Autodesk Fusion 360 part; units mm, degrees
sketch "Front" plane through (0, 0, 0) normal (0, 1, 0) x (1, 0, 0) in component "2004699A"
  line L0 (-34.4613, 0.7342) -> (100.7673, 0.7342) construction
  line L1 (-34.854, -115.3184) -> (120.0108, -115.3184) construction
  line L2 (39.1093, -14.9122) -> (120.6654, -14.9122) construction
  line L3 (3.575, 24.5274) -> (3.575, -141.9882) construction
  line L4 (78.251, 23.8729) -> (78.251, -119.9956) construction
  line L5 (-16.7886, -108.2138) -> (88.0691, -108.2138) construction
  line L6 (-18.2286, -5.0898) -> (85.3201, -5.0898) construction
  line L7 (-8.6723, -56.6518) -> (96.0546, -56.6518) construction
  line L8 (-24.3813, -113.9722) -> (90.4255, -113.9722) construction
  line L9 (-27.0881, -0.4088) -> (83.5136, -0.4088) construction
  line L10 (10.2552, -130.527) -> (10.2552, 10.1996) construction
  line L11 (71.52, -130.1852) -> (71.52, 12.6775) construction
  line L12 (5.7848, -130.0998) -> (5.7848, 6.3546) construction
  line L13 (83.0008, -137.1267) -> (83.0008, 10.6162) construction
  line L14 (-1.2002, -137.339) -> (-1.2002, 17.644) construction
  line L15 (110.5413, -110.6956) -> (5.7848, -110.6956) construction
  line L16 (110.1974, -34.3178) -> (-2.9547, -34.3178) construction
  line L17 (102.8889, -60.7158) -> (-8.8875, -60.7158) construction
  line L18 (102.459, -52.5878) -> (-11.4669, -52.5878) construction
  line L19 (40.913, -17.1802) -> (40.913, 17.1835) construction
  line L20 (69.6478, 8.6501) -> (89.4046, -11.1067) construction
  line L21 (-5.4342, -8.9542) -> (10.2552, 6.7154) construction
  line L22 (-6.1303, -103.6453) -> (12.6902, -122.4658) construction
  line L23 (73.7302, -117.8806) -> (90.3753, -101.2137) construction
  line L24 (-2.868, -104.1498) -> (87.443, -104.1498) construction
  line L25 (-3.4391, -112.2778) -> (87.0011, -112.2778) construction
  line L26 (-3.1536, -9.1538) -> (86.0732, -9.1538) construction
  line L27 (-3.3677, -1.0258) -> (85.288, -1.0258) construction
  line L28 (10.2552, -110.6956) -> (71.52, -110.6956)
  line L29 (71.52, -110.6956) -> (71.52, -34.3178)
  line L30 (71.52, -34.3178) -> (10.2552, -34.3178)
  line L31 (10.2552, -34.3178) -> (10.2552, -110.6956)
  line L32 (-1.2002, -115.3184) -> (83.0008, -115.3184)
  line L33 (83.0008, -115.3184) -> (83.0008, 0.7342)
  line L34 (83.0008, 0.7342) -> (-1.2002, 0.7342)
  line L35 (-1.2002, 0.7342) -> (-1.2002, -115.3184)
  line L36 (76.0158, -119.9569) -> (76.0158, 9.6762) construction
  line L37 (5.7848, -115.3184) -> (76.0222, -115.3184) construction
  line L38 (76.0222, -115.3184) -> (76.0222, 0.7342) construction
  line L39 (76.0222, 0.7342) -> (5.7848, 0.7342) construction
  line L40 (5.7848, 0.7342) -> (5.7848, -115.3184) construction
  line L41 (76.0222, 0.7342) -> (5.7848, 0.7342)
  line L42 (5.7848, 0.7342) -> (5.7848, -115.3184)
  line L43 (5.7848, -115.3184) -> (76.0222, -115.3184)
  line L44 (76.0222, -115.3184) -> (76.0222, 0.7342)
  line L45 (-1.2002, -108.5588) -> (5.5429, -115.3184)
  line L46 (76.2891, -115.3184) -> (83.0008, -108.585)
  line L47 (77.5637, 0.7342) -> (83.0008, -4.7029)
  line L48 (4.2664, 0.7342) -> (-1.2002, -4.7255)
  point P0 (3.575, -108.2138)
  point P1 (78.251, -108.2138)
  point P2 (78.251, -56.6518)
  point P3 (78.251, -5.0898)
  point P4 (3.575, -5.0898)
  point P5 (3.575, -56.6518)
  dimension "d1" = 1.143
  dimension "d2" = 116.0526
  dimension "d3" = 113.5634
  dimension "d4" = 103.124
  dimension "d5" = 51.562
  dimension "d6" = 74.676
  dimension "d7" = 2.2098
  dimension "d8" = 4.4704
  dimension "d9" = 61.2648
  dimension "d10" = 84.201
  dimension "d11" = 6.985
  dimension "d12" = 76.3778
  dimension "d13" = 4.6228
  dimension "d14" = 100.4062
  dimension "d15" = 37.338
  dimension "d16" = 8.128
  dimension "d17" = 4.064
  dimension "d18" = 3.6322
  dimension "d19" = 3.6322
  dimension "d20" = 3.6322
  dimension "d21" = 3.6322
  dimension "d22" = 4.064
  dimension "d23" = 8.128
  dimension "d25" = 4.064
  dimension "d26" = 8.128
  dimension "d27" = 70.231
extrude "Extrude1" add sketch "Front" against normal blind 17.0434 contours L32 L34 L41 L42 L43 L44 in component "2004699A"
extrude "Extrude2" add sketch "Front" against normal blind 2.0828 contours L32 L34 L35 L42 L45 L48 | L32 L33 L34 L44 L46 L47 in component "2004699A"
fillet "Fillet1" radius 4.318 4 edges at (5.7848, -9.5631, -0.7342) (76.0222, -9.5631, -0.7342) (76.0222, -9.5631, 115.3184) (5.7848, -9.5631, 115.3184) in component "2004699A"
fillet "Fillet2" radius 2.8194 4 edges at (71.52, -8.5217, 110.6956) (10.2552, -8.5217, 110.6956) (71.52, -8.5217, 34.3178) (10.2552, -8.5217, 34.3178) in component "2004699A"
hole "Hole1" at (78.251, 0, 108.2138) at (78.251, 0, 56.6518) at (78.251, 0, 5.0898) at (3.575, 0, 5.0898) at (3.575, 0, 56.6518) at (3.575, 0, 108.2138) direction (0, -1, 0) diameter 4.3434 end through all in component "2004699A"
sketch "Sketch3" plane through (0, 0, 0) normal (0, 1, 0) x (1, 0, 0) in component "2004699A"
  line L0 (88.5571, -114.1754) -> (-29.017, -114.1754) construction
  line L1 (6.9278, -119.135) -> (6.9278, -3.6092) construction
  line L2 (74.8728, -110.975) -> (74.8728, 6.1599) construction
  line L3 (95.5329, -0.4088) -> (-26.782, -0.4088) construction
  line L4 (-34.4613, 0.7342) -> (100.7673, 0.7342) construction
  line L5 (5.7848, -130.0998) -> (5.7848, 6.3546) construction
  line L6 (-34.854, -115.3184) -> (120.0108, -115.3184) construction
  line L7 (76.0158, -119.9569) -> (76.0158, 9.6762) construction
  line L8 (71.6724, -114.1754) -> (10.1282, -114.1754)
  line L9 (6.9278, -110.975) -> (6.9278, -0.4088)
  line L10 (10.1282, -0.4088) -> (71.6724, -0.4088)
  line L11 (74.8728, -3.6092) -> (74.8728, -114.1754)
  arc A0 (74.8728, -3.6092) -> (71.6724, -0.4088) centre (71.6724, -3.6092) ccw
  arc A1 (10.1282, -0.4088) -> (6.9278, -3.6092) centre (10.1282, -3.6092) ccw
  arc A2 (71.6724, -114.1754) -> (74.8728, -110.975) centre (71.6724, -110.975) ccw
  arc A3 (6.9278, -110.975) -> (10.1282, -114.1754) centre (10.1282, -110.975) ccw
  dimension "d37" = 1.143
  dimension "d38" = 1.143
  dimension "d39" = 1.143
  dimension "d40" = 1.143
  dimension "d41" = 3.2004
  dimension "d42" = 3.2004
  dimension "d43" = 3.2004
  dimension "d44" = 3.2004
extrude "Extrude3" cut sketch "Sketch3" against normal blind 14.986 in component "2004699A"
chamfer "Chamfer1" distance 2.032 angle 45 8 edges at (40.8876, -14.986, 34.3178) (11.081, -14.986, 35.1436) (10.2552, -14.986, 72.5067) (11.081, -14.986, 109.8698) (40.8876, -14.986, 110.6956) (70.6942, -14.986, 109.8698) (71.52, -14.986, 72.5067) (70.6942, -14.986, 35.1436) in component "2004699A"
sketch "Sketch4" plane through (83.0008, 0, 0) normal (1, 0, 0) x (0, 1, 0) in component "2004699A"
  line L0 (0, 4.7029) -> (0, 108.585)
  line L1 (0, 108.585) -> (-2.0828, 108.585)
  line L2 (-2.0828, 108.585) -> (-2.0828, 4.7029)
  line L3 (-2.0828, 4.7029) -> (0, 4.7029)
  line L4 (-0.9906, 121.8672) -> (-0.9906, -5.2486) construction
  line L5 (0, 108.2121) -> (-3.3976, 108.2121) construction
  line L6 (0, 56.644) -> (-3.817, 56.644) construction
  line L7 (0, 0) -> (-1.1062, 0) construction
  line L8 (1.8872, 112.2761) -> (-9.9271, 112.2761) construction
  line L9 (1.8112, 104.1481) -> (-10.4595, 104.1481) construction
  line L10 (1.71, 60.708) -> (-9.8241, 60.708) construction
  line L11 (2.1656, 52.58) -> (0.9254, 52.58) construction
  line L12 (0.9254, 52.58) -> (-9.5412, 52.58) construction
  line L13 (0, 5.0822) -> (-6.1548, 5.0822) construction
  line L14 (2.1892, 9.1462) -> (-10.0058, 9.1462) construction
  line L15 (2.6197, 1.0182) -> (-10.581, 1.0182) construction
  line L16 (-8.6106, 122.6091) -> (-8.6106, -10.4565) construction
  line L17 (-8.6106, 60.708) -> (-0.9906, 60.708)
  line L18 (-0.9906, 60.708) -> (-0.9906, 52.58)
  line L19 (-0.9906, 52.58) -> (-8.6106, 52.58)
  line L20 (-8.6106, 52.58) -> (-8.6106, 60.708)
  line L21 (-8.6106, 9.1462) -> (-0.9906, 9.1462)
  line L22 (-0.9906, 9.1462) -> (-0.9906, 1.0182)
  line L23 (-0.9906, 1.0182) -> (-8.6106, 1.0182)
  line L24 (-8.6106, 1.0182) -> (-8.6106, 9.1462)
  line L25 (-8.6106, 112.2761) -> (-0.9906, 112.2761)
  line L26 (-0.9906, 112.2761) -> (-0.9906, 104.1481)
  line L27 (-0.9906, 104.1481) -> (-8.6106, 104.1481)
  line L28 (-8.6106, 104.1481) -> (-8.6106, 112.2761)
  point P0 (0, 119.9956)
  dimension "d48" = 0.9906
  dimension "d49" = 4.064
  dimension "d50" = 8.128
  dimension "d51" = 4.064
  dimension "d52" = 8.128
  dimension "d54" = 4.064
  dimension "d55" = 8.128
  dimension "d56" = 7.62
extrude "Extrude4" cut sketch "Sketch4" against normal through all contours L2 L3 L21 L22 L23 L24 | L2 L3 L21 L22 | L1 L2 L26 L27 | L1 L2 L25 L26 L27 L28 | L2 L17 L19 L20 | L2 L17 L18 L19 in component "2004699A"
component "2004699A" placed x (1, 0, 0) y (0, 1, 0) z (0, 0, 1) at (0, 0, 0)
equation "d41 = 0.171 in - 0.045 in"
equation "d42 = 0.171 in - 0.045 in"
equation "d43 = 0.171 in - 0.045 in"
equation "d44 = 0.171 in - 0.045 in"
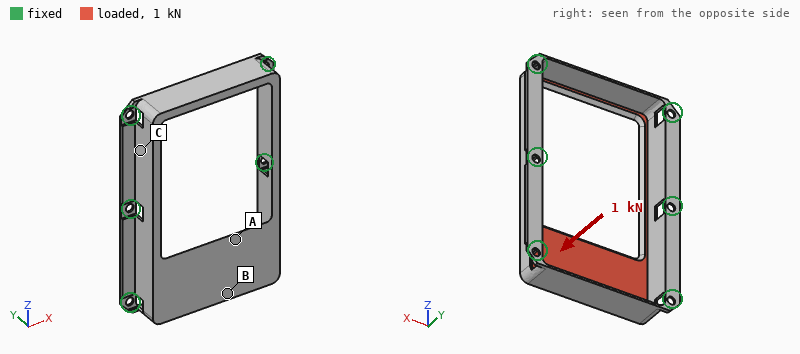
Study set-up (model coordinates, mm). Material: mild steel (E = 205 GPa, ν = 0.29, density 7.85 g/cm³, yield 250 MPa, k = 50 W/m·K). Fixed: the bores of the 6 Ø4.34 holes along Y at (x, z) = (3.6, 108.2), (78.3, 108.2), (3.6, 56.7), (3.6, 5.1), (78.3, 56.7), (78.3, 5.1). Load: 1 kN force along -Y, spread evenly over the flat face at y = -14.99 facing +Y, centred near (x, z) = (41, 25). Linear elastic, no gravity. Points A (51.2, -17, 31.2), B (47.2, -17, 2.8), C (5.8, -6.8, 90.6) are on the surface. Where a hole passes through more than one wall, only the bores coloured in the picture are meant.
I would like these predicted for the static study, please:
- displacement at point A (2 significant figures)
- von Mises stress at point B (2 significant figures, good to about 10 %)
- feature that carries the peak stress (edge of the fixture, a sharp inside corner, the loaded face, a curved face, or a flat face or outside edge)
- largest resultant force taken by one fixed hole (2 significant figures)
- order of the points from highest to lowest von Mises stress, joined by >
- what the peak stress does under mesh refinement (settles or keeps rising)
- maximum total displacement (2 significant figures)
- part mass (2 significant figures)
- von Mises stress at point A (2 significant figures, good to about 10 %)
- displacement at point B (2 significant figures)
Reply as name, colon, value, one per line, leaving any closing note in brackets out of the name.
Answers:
displacement at point A: 0.19 mm
von Mises stress at point B: 39 MPa
feature that carries the peak stress: edge of the fixture
largest resultant force taken by one fixed hole: 410 N
order of the points from highest to lowest von Mises stress, joined by >: A > B > C
what the peak stress does under mesh refinement: keeps rising
maximum total displacement: 0.23 mm
part mass: 120 g
von Mises stress at point A: 96 MPa
displacement at point B: 0.042 mm
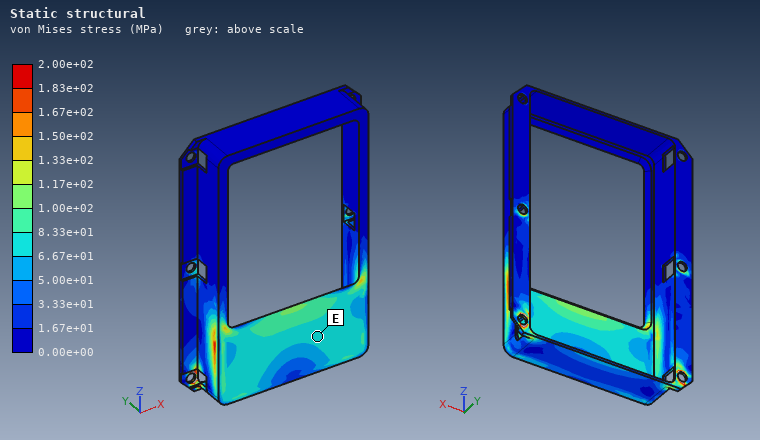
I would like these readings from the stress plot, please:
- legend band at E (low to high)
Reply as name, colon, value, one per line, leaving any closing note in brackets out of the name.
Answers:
legend band at E: 6.67e+01 to 8.33e+01 MPa
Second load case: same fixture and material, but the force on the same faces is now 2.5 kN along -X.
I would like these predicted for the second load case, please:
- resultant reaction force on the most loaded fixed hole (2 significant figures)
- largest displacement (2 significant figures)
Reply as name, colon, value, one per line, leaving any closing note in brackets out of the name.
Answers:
resultant reaction force on the most loaded fixed hole: 1.3 kN
largest displacement: 62 µm
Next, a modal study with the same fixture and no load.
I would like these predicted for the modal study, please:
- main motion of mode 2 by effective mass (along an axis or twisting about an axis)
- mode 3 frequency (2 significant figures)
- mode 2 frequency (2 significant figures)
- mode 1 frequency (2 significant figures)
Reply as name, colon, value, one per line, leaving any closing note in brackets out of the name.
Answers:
main motion of mode 2 by effective mass: along Y
mode 3 frequency: 3200 Hz
mode 2 frequency: 2100 Hz
mode 1 frequency: 2000 Hz
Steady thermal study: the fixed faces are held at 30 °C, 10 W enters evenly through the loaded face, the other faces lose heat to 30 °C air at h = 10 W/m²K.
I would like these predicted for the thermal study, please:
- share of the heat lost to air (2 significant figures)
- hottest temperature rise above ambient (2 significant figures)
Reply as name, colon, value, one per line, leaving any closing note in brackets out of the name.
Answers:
share of the heat lost to air: 33 %
hottest temperature rise above ambient: 47 K
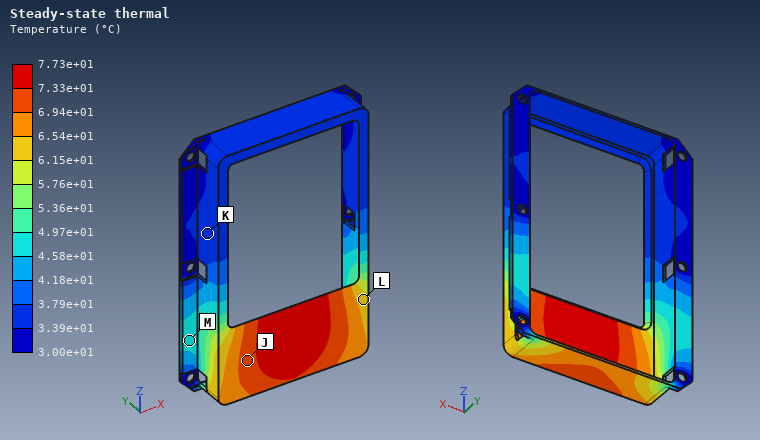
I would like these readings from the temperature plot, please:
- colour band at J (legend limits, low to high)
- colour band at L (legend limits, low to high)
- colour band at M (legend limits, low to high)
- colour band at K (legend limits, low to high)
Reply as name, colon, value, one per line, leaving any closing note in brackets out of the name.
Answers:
colour band at J: 6.94e+01 to 7.33e+01 °C
colour band at L: 6.15e+01 to 6.54e+01 °C
colour band at M: 4.58e+01 to 4.97e+01 °C
colour band at K: 3.39e+01 to 3.79e+01 °C
